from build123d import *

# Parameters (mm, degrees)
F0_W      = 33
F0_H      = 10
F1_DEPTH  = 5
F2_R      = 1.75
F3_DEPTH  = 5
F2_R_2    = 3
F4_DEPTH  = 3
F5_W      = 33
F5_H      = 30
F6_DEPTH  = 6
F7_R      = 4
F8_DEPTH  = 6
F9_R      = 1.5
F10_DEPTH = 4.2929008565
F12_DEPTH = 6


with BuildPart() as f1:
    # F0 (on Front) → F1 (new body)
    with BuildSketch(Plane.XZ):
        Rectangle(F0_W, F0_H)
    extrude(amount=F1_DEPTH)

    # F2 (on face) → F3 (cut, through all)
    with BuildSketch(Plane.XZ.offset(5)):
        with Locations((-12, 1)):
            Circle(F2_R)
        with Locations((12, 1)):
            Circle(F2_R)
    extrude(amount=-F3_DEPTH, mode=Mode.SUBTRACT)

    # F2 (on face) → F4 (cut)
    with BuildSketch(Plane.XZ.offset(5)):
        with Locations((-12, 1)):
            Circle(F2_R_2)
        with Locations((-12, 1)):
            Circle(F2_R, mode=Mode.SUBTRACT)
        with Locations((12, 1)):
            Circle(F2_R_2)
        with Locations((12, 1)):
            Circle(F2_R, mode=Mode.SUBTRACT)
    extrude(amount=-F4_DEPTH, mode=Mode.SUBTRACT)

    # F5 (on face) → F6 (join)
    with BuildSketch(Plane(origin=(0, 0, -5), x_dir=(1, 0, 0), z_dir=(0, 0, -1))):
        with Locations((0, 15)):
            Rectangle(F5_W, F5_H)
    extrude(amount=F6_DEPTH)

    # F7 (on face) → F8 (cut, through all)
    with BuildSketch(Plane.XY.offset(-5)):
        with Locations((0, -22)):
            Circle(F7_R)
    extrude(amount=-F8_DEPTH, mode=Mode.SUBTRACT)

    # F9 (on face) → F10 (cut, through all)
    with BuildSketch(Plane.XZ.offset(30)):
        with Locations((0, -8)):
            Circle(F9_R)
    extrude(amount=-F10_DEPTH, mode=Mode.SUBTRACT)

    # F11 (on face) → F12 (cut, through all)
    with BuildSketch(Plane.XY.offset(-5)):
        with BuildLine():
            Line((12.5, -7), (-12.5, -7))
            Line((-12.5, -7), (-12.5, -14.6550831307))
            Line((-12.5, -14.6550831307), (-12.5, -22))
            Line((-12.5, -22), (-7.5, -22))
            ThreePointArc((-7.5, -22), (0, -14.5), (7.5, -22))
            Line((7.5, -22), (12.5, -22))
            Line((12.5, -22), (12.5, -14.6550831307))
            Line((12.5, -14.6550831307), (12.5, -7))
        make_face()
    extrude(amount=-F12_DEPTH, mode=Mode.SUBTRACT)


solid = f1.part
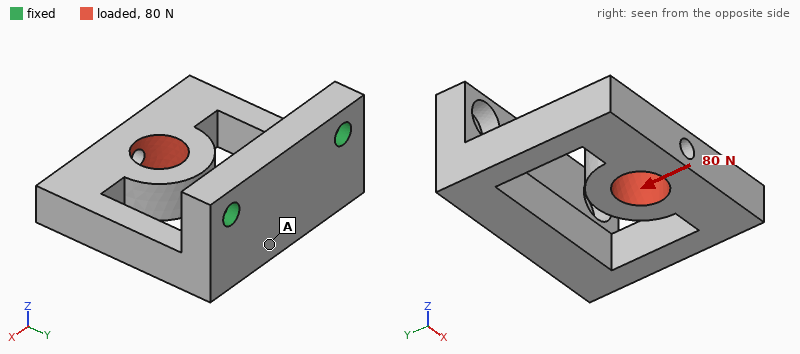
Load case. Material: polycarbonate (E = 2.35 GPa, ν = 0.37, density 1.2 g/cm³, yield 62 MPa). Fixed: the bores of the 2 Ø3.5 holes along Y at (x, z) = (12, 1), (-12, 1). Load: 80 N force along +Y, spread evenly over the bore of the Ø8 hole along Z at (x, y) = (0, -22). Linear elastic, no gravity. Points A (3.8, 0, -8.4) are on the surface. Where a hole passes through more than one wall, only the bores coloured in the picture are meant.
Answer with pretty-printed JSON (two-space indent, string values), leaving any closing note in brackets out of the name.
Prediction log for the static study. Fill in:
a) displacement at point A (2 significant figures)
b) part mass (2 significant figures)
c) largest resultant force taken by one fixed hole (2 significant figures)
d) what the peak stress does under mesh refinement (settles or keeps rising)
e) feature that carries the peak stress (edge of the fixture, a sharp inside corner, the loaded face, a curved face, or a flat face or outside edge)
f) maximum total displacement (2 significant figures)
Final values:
{
  "displacement at point A": "0.12 mm",
  "part mass": "6.4 g",
  "largest resultant force taken by one fixed hole": "41 N",
  "what the peak stress does under mesh refinement": "keeps rising",
  "feature that carries the peak stress": "edge of the fixture",
  "maximum total displacement": "0.52 mm"
}
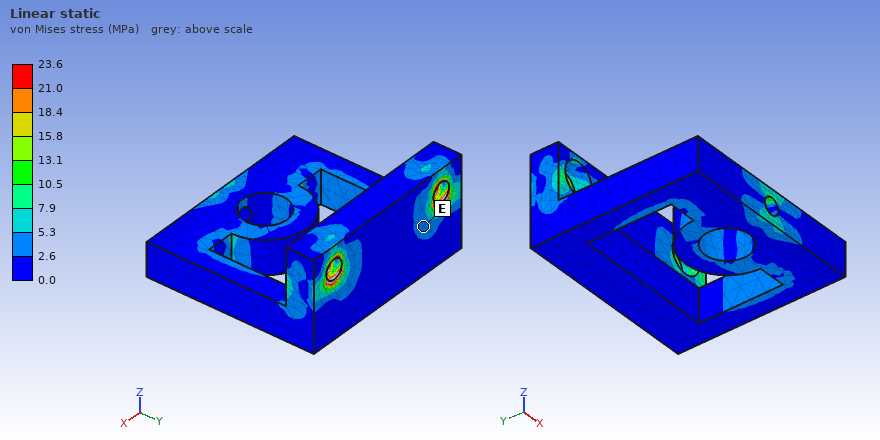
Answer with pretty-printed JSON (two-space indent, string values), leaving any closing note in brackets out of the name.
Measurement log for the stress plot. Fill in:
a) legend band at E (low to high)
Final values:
{
  "legend band at E": "2.6 to 5.3 MPa"
}
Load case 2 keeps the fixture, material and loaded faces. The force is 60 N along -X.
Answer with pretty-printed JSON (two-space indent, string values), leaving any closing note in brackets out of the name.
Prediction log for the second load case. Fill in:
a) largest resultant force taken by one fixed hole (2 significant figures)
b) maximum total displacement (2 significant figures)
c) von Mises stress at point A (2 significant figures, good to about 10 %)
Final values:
{
  "largest resultant force taken by one fixed hole": "61 N",
  "maximum total displacement": "0.45 mm",
  "von Mises stress at point A": "2.2 MPa"
}
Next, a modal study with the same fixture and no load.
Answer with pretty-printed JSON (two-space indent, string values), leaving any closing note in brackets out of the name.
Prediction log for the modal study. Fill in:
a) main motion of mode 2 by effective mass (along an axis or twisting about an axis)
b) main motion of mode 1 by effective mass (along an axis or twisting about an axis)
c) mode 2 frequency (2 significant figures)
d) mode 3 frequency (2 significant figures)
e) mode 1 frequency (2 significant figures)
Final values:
{
  "main motion of mode 2 by effective mass": "along X",
  "main motion of mode 1 by effective mass": "along Z",
  "mode 2 frequency": "1200 Hz",
  "mode 3 frequency": "1900 Hz",
  "mode 1 frequency": "610 Hz"
}
